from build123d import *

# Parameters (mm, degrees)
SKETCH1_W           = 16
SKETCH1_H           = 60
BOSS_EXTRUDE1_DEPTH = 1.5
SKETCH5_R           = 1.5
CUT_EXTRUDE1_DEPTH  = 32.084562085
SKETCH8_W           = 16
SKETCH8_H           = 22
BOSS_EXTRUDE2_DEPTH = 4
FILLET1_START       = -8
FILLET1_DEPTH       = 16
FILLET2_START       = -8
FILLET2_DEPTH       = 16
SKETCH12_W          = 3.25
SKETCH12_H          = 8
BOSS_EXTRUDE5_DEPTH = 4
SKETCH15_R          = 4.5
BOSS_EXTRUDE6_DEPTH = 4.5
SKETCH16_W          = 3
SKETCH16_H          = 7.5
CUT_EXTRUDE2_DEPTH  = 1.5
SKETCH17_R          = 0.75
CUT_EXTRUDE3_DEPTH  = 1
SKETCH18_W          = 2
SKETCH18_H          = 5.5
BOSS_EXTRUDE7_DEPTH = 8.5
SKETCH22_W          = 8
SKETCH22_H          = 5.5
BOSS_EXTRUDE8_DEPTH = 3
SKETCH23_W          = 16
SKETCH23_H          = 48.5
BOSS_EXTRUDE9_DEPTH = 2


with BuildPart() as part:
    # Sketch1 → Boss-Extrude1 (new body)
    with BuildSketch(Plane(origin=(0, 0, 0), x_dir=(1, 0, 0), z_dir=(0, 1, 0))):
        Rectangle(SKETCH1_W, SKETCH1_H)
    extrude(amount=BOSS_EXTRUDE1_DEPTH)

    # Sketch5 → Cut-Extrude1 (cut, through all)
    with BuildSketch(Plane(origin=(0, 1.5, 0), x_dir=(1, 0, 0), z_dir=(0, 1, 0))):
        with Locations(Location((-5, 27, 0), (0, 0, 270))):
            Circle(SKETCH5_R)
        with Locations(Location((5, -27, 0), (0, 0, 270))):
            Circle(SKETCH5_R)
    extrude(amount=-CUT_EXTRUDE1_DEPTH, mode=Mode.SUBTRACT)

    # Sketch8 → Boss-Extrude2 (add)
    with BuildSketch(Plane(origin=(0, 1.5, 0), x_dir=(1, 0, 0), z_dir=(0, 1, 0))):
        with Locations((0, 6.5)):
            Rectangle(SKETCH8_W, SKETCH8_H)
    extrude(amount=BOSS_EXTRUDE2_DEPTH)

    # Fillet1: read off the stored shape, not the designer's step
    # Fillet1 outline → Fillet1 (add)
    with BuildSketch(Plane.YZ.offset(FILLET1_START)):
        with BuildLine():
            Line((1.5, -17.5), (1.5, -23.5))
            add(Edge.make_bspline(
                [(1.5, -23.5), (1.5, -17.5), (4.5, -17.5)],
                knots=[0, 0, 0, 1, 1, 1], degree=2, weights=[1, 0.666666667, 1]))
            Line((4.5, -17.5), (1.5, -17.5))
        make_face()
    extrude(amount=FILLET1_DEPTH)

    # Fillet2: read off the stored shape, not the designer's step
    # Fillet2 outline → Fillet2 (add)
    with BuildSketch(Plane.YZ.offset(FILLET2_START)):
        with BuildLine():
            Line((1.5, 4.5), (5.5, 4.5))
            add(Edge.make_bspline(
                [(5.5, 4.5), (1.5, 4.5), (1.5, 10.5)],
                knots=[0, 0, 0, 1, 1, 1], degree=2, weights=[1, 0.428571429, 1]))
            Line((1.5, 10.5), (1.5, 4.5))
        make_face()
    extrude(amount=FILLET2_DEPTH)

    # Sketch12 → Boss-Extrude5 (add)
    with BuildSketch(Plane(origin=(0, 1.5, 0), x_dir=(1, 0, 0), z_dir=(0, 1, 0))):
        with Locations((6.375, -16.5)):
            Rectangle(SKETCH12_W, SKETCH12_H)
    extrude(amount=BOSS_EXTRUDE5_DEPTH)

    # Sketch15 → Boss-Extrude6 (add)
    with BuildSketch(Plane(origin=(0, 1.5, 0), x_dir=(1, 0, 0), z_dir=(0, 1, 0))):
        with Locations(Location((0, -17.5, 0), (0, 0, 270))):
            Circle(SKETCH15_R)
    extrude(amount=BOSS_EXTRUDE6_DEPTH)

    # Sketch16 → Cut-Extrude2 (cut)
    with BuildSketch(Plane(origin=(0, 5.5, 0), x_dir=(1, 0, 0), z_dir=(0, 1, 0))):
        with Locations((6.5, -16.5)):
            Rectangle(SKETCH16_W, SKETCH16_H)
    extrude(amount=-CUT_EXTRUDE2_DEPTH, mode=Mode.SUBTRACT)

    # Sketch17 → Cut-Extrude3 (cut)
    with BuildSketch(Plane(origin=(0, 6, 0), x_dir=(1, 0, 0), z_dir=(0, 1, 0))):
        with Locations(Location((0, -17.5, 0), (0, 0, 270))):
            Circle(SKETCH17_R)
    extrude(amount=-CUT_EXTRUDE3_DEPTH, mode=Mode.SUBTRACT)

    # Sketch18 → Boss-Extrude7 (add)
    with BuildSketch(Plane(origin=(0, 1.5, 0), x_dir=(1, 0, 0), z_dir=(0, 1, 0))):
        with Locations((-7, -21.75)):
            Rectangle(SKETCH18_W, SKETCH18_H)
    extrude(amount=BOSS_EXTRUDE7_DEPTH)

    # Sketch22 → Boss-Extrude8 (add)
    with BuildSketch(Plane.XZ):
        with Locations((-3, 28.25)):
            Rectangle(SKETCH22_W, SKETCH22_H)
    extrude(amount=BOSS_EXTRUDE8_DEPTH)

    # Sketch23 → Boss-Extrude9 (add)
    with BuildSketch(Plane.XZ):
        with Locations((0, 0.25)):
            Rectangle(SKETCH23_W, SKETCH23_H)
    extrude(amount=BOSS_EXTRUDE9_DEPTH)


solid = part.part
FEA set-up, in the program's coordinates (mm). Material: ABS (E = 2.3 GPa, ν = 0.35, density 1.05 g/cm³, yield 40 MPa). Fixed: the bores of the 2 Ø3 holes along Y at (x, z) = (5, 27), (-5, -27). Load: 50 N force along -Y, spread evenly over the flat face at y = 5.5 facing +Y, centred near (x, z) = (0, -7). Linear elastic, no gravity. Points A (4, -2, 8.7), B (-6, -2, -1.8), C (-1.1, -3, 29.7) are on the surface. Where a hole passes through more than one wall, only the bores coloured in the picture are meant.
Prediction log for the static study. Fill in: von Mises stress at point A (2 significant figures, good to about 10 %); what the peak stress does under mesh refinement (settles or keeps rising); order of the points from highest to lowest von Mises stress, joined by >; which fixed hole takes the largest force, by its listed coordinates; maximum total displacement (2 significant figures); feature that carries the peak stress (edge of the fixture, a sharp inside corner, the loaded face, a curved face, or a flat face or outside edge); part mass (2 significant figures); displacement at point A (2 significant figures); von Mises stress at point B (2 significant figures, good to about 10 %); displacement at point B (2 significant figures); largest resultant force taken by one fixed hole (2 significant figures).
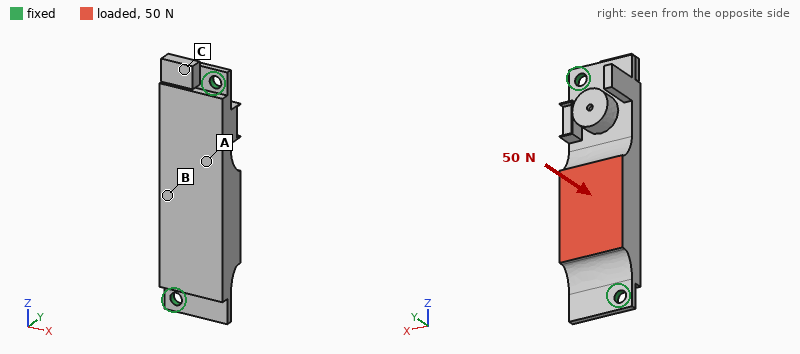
6.9 MPa
keeps rising
A > B > C
(-5, -27)
0.27 mm
edge of the fixture
5.4 g
0.23 mm
2.9 MPa
0.17 mm
34 N
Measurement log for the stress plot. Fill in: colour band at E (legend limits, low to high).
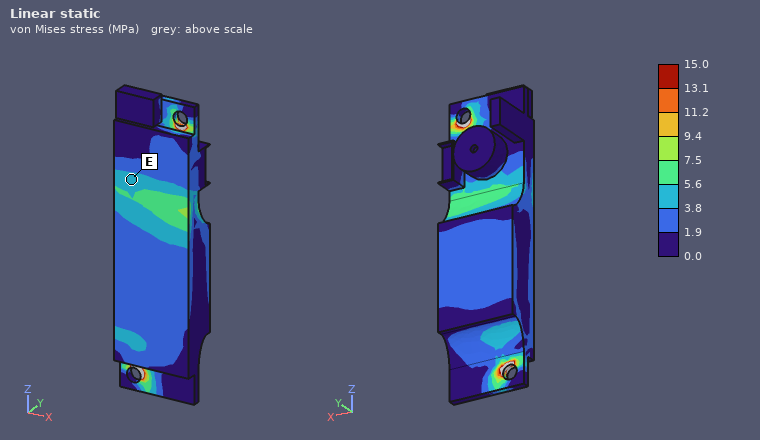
3.8 to 5.6 MPa
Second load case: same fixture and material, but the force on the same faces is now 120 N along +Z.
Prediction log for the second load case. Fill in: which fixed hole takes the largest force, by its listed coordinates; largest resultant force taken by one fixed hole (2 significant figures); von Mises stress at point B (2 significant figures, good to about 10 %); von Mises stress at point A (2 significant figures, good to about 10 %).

(-5, -27)
78 N
1.5 MPa
3.6 MPa
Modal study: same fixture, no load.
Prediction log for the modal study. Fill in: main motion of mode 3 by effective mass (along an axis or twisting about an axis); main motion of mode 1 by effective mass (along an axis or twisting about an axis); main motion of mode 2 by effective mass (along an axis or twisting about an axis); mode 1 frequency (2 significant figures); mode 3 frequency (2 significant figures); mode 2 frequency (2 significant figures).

along X
twisting about Z
along Y
1200 Hz
2800 Hz
1200 Hz
